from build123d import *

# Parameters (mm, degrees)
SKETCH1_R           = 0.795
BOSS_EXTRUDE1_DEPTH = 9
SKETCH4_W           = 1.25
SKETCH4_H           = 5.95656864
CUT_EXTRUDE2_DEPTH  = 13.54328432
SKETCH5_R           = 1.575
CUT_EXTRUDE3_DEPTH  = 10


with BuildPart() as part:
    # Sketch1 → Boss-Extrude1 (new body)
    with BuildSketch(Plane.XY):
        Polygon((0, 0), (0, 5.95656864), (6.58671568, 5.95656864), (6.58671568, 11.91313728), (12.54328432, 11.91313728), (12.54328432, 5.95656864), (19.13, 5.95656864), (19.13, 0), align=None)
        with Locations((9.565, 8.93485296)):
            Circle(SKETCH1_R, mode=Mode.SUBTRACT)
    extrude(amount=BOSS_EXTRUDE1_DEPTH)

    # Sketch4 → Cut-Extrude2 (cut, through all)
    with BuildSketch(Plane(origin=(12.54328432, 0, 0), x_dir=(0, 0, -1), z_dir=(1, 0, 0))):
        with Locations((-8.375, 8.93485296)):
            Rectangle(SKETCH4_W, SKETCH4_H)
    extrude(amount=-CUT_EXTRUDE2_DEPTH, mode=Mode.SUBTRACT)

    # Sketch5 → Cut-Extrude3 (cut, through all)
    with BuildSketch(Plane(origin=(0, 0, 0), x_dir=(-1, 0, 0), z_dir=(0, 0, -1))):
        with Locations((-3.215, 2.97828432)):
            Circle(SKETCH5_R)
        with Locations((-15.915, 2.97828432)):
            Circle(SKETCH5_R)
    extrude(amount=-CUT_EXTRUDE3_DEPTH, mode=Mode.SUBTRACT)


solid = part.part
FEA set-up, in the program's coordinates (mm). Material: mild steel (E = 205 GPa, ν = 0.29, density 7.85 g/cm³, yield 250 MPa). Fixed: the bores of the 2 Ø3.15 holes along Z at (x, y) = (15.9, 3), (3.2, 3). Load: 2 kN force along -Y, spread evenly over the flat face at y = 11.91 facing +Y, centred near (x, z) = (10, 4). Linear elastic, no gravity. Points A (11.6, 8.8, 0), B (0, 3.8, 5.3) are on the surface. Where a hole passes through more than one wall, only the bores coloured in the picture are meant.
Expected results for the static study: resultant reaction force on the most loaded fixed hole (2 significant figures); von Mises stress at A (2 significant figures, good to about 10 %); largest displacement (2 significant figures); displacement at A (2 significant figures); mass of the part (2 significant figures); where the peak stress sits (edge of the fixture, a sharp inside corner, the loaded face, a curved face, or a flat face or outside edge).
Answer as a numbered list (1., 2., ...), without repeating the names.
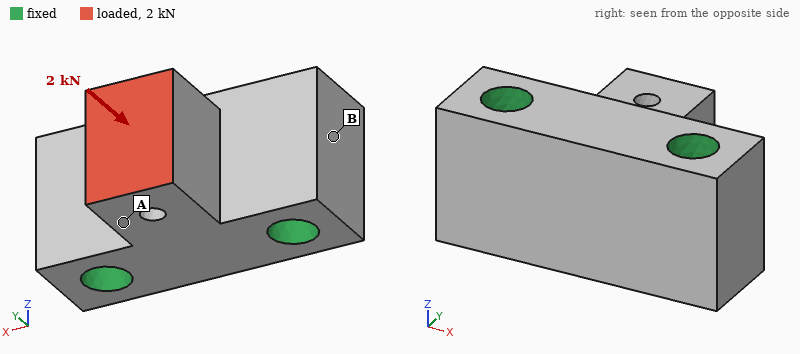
1. 1.0 kN
2. 46 MPa
3. 3.3 µm
4. 2.4 µm
5. 9.0 g
6. a curved face
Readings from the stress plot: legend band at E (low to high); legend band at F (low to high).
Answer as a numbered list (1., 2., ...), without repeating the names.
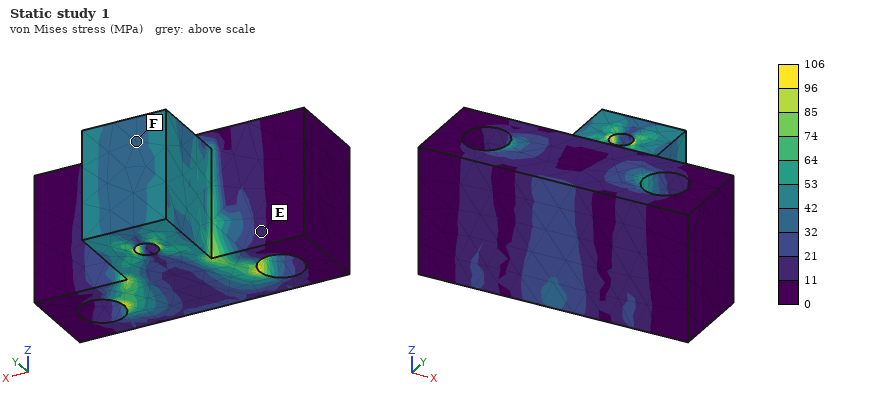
1. 11 to 21 MPa
2. 32 to 42 MPa
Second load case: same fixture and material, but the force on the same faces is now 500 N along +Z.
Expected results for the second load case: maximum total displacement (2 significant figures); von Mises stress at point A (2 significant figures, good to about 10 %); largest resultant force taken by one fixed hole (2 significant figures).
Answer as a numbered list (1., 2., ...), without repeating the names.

1. 5.3 µm
2. 30 MPa
3. 250 N
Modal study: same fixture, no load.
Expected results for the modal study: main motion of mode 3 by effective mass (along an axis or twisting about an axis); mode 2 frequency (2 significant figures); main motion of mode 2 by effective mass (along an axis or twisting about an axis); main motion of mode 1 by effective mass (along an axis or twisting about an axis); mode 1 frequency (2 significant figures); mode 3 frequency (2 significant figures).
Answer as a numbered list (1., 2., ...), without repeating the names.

1. along Y
2. 63 kHz
3. along X
4. along Z
5. 52 kHz
6. 92 kHz
